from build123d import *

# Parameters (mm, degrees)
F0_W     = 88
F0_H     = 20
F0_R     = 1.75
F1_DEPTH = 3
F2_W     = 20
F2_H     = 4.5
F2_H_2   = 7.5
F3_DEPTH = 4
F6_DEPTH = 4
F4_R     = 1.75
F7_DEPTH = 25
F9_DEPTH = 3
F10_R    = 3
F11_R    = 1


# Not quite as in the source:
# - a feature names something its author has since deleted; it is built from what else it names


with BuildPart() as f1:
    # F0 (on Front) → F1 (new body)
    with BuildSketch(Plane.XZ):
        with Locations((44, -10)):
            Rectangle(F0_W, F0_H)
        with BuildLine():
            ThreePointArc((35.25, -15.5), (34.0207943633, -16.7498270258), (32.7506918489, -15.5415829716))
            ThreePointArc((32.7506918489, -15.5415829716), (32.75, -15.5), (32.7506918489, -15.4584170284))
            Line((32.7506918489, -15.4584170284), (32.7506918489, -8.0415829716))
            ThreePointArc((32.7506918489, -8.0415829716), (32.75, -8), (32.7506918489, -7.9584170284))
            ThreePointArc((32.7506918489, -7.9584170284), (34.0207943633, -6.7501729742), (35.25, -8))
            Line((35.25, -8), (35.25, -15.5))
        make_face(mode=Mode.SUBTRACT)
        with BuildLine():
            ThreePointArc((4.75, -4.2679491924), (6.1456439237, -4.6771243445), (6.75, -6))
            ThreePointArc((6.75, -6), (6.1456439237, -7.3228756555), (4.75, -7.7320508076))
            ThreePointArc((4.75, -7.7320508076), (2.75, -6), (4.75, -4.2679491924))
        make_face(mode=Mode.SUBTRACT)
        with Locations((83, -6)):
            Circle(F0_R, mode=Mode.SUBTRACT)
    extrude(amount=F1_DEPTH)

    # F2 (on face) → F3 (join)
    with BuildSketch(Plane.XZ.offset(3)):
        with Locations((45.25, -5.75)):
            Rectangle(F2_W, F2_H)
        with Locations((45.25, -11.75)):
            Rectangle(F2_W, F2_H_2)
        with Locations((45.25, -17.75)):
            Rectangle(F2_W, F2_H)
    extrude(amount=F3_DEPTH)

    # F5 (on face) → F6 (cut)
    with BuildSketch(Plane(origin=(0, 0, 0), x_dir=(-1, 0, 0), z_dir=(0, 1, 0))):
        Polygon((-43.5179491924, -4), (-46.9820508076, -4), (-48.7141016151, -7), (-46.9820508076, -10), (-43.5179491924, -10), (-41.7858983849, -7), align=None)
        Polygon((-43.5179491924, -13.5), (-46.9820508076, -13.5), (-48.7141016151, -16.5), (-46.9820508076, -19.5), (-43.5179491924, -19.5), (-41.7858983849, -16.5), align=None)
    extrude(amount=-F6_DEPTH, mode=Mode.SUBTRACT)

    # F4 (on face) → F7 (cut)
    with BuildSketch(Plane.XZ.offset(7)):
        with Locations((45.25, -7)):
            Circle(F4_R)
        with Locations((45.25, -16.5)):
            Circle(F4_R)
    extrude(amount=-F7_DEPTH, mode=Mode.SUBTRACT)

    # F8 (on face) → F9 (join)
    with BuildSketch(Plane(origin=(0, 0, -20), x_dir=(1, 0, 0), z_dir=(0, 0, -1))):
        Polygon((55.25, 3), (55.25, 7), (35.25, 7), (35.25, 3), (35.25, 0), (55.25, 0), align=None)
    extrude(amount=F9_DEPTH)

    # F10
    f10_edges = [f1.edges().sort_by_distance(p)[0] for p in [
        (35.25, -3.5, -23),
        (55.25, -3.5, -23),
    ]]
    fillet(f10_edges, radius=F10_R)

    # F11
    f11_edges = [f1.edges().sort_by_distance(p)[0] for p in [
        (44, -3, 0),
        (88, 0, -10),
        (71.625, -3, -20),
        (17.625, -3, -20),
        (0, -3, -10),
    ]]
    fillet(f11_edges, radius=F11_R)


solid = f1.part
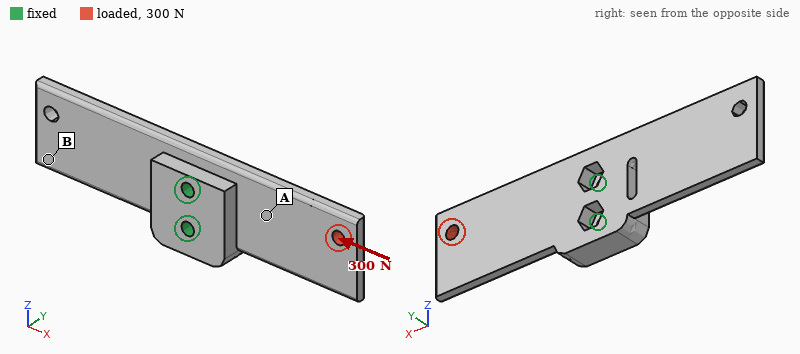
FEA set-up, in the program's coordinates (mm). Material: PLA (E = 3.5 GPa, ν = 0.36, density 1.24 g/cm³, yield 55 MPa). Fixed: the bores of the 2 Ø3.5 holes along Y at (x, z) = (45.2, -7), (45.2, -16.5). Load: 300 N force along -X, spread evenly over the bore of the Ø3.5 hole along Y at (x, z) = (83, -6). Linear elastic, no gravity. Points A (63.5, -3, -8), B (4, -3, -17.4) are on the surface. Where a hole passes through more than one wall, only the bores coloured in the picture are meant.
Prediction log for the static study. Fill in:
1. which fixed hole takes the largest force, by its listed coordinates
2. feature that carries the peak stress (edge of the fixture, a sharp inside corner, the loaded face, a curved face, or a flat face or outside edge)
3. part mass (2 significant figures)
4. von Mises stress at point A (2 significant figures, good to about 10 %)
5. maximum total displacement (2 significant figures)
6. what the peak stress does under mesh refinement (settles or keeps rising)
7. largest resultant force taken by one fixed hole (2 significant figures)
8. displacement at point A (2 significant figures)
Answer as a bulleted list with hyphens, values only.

- (45.2, -7)
- edge of the fixture
- 8.1 g
- 6.5 MPa
- 0.50 mm
- keeps rising
- 300 N
- 0.18 mm
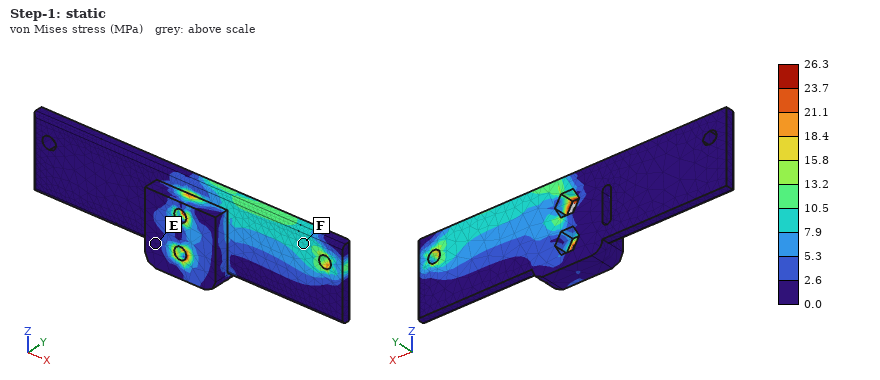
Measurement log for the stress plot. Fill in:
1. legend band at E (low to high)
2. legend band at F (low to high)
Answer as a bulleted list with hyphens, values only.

- 0.0 to 2.6 MPa
- 7.9 to 10.5 MPa
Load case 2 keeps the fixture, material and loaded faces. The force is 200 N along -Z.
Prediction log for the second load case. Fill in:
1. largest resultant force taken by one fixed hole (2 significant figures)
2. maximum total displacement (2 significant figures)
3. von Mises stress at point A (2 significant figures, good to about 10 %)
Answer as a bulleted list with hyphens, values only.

- 650 N
- 0.85 mm
- 9.9 MPa
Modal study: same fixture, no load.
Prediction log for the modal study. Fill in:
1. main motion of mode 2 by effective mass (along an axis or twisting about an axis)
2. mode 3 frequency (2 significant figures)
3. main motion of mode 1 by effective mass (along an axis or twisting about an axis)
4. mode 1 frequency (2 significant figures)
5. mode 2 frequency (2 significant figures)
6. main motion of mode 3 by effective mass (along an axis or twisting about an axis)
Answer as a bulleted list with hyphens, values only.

- along Y
- 2000 Hz
- along Y
- 460 Hz
- 640 Hz
- twisting about Y
